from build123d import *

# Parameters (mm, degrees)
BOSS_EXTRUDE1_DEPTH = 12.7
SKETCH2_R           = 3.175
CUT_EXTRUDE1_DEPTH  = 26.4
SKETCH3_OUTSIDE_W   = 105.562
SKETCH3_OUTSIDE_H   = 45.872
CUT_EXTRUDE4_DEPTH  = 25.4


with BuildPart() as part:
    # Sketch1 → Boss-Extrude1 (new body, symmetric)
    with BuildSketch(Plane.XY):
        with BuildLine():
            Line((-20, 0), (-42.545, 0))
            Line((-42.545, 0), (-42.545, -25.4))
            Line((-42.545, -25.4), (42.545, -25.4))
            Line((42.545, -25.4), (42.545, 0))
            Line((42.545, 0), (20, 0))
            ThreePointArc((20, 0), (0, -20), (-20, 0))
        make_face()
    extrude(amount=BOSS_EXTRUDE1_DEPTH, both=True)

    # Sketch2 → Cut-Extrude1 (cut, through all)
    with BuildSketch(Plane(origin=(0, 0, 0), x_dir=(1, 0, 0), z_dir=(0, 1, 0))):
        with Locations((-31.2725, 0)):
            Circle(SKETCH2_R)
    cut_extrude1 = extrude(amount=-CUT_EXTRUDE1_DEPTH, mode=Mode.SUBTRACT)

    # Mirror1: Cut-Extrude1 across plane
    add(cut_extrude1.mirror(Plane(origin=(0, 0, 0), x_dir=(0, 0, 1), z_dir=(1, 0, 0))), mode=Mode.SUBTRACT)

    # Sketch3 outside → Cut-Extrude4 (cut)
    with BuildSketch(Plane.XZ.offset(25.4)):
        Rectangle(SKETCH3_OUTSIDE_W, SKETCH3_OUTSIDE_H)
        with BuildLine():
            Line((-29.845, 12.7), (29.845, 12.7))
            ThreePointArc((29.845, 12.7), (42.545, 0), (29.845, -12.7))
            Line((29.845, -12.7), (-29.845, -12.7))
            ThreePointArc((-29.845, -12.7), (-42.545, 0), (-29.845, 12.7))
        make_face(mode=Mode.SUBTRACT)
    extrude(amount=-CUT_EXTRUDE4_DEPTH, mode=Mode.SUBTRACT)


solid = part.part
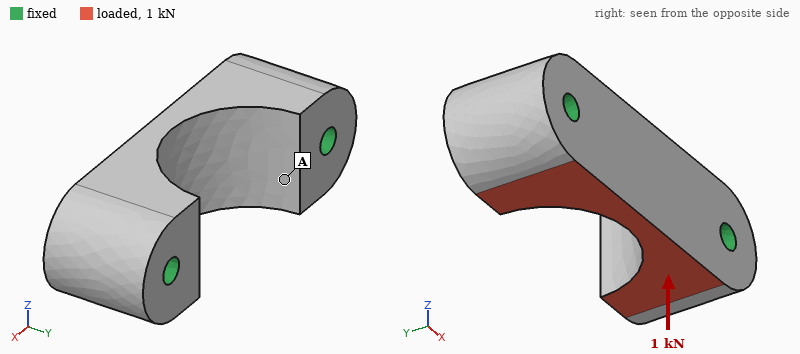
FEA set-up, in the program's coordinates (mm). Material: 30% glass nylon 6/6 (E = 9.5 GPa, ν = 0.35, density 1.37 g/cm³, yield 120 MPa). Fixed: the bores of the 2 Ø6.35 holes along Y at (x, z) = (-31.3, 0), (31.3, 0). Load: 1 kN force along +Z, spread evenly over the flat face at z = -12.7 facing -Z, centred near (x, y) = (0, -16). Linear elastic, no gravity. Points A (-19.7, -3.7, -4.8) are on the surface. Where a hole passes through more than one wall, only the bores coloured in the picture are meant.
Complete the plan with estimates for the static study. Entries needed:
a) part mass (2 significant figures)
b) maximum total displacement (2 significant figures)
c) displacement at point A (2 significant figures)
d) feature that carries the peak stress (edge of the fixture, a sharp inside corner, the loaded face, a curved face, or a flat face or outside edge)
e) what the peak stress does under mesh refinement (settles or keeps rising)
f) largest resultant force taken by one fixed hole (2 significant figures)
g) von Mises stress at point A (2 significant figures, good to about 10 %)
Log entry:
46 g
16 µm
5.0 µm
edge of the fixture
keeps rising
500 N
1.2 MPa
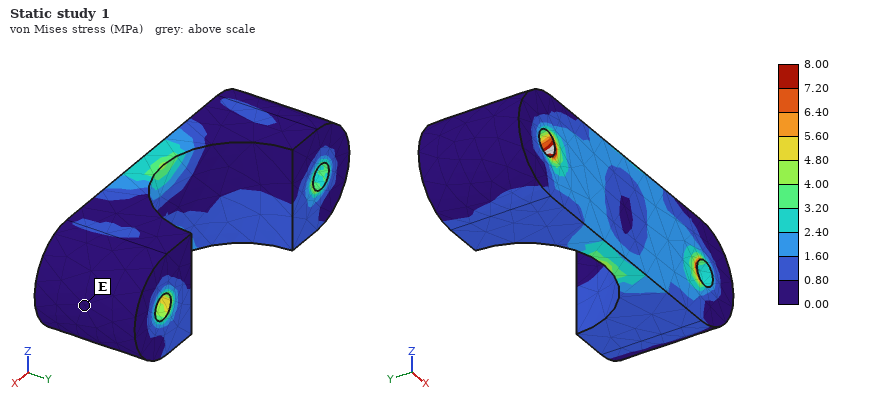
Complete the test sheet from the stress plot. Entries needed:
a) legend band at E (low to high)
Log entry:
0.00 to 0.80 MPa
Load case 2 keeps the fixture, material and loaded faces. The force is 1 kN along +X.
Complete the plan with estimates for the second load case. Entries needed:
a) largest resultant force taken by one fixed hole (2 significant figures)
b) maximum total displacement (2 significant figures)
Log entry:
520 N
7.2 µm
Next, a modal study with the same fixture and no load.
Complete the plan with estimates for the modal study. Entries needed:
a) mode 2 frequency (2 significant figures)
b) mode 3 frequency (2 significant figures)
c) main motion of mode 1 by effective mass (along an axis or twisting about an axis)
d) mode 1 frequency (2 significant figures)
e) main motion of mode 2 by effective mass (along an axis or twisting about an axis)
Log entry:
12 kHz
16 kHz
along Z
9100 Hz
along Y
